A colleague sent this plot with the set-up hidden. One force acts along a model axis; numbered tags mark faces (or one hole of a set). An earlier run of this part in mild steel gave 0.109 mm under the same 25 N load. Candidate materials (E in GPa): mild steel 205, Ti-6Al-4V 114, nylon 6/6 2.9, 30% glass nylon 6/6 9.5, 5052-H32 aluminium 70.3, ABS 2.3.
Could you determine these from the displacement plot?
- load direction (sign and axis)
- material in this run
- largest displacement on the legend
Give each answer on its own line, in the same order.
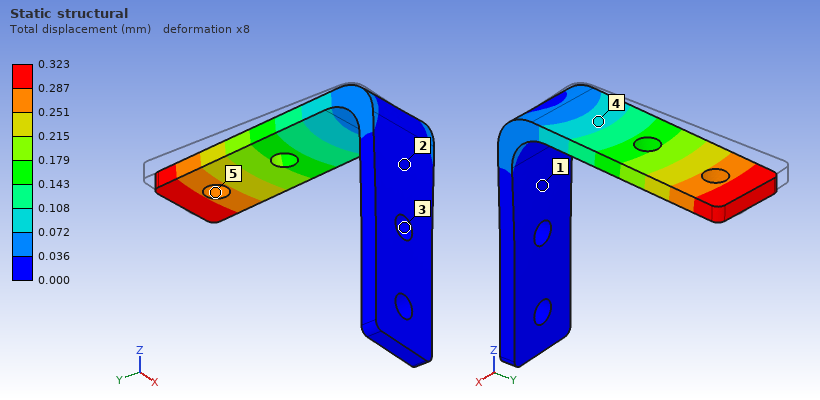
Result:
+X
5052-H32 aluminium
0.323 mm
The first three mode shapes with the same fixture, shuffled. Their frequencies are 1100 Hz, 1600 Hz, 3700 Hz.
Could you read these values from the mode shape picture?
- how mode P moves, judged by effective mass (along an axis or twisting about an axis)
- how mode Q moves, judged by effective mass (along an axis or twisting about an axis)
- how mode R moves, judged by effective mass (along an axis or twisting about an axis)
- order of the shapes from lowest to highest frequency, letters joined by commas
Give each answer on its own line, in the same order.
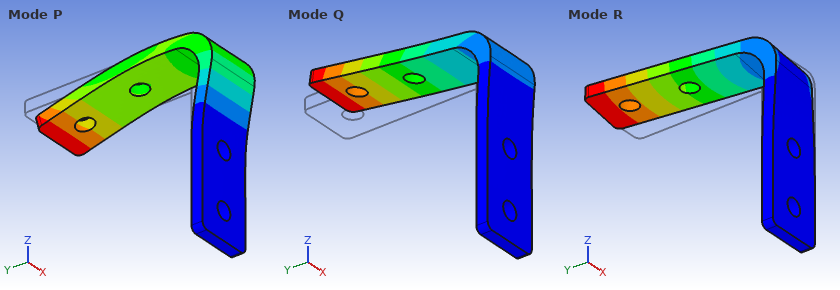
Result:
along Y
along Z
along X
Q, R, P
